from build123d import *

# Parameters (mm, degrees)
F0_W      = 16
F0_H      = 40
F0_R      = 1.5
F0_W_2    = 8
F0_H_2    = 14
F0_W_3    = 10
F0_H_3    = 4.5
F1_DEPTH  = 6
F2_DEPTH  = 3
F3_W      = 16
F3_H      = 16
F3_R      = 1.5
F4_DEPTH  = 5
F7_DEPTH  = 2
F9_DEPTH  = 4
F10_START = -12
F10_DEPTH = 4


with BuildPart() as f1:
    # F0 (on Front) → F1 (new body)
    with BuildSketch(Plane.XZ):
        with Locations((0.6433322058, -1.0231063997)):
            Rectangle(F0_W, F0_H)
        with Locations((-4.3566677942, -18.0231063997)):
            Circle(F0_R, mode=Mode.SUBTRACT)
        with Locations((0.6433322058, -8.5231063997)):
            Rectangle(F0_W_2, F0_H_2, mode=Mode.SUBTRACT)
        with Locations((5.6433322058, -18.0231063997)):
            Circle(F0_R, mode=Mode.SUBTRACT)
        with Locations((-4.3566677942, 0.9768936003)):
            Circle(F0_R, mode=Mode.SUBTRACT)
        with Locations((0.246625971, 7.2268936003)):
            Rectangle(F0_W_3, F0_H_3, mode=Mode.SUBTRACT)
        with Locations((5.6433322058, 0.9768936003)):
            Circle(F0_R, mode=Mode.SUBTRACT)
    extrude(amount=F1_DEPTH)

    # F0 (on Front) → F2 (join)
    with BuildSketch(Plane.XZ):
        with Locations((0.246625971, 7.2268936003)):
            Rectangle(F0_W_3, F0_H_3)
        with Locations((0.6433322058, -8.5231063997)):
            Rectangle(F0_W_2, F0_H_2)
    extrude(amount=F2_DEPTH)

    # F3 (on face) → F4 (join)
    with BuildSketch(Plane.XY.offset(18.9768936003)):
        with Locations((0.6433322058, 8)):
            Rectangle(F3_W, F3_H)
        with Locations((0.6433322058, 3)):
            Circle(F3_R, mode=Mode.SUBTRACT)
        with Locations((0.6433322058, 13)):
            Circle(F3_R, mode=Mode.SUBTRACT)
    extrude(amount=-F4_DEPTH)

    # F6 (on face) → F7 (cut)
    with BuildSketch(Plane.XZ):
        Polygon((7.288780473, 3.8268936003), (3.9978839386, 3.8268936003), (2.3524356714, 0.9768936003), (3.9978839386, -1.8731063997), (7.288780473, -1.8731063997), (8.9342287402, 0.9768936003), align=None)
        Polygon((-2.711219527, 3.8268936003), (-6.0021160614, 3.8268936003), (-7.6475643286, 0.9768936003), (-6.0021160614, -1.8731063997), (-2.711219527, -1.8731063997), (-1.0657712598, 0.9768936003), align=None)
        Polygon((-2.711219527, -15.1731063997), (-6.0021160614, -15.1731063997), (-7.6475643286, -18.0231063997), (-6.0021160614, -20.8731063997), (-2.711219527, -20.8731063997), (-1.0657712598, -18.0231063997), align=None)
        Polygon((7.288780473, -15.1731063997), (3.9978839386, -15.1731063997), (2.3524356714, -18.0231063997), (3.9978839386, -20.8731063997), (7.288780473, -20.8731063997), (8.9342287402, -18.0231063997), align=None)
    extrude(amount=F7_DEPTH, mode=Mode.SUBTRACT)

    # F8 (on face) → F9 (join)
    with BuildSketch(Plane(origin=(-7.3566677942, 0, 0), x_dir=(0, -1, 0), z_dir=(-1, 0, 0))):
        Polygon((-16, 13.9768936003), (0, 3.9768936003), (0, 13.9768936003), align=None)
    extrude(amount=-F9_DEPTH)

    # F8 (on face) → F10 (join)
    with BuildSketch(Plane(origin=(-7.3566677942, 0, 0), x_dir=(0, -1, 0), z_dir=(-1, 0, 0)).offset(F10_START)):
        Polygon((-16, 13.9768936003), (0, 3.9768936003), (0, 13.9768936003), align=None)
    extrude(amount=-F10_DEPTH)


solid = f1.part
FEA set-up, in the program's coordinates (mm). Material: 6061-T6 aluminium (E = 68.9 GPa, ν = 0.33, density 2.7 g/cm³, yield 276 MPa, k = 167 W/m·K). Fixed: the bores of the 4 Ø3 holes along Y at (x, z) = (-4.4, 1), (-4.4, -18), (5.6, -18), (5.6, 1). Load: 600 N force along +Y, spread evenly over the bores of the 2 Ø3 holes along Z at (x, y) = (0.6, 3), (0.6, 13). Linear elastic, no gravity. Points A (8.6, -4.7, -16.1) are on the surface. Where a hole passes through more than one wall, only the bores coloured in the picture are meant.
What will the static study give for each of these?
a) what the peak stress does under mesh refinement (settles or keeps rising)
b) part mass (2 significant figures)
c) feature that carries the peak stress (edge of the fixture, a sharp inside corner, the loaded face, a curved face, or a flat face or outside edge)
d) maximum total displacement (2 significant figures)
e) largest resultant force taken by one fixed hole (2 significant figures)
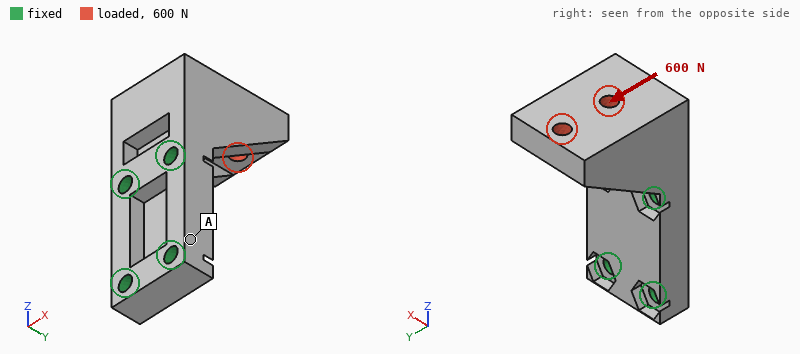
keeps rising
13 g
edge of the fixture
0.16 mm
380 N
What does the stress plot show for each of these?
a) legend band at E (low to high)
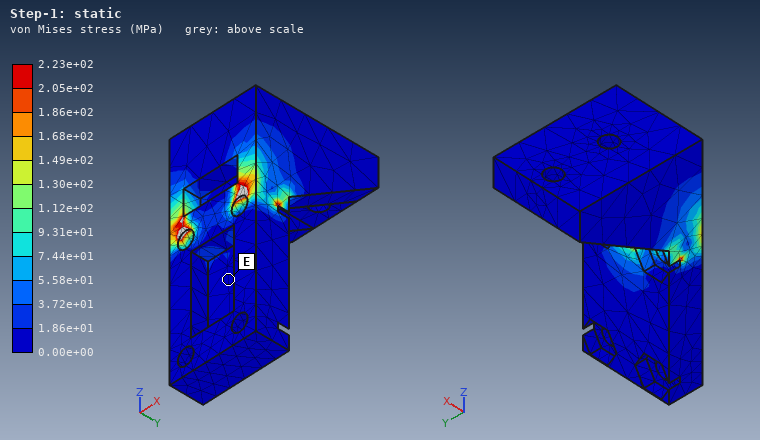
0.00e+00 to 1.86e+01 MPa
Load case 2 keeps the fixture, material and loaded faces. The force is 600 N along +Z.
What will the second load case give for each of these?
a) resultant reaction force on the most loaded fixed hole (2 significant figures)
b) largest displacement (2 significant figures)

200 N
0.14 mm
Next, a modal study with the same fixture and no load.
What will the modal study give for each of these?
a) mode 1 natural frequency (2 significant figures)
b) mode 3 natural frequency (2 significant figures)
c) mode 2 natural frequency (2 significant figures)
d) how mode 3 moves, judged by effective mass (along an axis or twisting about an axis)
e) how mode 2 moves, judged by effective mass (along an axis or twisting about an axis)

4400 Hz
15 kHz
9500 Hz
along X
along X
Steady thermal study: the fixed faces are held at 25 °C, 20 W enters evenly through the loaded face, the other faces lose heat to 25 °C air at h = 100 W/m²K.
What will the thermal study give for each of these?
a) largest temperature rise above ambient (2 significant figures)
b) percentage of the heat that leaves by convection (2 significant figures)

26 K
14 %
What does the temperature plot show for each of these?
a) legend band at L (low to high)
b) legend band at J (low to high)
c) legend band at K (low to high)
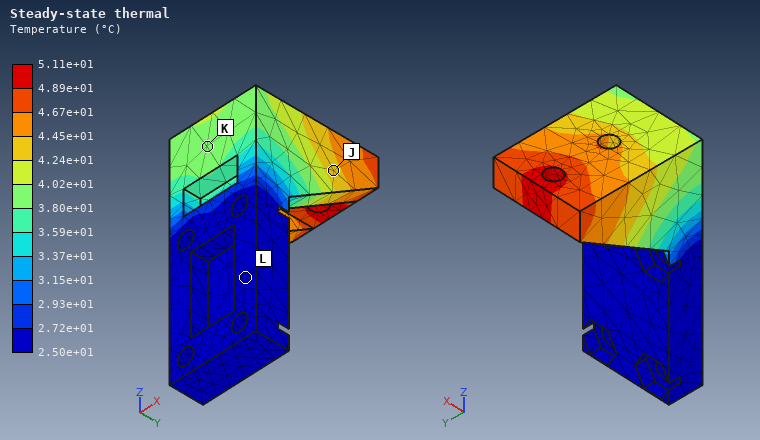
2.50e+01 to 2.72e+01 °C
4.24e+01 to 4.45e+01 °C
3.80e+01 to 4.02e+01 °C
